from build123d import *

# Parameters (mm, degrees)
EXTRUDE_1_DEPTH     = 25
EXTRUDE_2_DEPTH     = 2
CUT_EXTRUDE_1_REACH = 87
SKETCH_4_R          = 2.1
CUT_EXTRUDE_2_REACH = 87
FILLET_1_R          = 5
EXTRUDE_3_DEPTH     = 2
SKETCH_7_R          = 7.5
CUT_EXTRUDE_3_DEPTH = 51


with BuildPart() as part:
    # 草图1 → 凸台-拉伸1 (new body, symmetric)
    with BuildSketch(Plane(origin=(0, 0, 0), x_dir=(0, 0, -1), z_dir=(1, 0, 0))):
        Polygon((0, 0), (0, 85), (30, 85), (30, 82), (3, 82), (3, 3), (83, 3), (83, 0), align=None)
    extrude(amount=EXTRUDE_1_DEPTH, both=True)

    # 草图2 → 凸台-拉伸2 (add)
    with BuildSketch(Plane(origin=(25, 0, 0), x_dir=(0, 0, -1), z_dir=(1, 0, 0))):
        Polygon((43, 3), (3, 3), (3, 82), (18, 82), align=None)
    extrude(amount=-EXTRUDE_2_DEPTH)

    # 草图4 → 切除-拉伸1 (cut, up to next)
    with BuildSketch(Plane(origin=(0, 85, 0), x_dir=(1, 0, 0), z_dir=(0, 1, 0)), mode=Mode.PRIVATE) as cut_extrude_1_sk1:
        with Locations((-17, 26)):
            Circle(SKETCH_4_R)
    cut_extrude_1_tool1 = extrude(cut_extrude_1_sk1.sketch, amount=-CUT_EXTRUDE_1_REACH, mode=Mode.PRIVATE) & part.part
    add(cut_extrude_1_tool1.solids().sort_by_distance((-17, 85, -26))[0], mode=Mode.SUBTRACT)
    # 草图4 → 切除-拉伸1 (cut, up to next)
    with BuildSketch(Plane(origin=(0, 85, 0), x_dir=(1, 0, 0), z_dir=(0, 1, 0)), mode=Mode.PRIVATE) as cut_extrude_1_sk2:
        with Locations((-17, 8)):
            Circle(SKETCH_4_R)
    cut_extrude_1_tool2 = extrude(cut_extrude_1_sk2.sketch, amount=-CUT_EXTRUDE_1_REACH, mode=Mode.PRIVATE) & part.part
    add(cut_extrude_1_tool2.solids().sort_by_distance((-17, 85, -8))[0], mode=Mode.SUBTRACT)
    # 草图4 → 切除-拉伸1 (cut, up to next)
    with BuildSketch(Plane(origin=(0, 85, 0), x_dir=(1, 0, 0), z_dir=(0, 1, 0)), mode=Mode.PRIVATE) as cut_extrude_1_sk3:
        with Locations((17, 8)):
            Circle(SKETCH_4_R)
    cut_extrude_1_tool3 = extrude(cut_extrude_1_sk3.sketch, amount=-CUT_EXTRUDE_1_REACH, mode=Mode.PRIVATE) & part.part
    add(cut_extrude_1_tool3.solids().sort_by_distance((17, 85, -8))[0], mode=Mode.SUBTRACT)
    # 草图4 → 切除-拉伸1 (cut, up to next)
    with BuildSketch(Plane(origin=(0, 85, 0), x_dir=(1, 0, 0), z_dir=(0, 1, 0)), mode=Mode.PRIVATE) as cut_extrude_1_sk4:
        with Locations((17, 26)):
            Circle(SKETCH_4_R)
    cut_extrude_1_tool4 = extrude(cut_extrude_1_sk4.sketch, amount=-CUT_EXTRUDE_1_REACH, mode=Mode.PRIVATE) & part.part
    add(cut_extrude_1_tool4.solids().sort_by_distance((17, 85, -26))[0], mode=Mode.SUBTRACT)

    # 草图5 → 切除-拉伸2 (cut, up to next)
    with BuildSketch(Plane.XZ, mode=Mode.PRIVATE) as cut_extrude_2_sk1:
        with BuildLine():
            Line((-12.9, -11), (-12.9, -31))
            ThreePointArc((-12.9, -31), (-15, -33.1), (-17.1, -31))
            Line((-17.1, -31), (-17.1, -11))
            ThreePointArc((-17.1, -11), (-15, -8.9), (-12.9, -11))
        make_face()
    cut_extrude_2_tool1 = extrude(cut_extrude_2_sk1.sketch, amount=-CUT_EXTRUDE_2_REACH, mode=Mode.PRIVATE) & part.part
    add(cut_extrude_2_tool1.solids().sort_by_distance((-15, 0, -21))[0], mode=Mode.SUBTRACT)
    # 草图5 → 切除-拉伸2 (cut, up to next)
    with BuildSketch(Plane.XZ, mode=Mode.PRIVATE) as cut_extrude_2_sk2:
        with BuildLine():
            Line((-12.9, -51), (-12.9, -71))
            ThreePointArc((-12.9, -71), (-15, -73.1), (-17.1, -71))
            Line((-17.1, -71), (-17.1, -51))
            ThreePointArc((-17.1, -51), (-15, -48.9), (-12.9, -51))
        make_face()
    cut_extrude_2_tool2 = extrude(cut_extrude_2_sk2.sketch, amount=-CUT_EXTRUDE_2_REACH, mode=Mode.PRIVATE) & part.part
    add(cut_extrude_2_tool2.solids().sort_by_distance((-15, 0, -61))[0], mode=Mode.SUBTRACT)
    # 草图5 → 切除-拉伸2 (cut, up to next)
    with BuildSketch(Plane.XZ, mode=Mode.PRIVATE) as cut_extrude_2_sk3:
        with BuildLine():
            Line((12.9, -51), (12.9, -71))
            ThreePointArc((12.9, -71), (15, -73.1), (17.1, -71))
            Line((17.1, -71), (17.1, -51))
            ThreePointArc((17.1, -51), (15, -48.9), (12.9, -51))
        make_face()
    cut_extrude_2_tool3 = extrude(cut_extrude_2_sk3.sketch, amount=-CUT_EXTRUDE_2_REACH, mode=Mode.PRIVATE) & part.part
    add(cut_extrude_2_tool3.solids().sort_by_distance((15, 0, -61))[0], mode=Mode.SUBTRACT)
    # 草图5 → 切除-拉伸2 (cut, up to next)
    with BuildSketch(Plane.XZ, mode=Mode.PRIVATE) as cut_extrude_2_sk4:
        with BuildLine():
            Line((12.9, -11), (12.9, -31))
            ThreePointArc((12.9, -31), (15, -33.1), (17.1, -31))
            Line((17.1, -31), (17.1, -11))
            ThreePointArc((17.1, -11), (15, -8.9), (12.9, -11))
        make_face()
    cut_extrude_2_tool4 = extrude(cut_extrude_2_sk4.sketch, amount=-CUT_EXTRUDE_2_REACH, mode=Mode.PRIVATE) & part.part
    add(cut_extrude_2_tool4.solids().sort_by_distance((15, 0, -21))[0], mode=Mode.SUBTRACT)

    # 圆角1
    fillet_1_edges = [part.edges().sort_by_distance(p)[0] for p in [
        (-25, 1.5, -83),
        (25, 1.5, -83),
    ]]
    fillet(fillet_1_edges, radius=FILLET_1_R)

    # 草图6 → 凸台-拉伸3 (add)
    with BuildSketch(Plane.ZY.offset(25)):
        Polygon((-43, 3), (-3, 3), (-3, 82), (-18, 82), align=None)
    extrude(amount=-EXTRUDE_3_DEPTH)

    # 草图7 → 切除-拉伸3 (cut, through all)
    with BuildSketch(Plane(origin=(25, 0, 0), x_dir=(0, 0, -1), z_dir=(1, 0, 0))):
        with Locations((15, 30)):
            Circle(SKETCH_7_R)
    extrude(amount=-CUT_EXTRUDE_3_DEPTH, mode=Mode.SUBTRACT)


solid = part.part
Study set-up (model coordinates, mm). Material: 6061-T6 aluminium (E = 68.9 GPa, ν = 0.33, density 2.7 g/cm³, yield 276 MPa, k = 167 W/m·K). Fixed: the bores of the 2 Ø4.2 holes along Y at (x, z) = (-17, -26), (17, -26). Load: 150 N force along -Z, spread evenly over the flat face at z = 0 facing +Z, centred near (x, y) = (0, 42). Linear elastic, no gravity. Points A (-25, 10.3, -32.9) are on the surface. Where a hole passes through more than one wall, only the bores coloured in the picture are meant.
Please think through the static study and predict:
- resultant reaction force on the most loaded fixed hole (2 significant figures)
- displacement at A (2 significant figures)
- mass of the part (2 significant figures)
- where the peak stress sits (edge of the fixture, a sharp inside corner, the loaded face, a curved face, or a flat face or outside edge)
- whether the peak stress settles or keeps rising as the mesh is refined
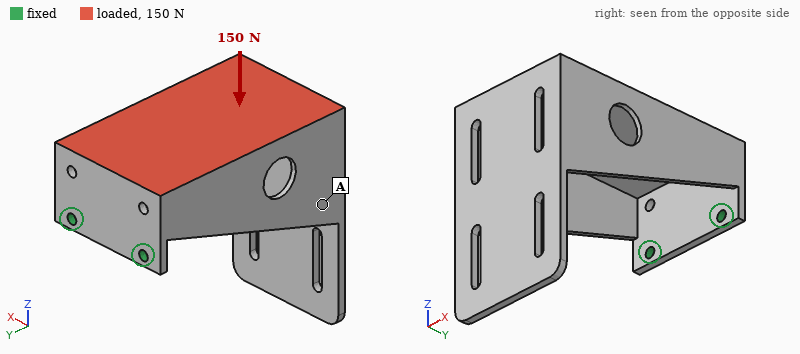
77 N
0.92 mm
96 g
edge of the fixture
keeps rising
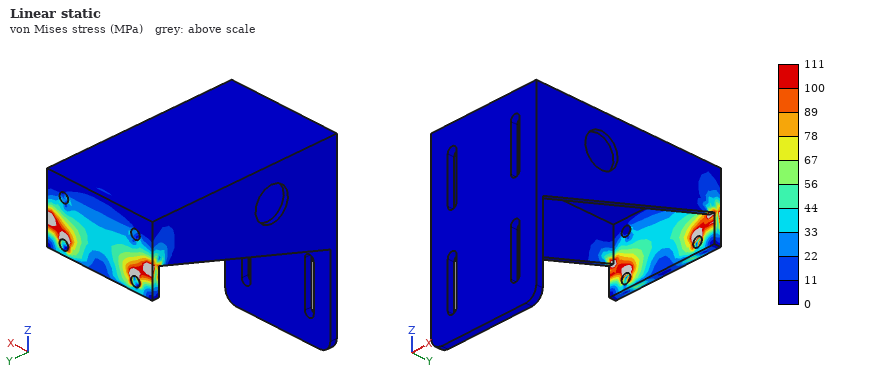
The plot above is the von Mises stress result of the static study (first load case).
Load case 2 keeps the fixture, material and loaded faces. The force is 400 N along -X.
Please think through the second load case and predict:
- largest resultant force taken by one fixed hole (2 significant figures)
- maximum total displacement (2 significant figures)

520 N
1.0 mm
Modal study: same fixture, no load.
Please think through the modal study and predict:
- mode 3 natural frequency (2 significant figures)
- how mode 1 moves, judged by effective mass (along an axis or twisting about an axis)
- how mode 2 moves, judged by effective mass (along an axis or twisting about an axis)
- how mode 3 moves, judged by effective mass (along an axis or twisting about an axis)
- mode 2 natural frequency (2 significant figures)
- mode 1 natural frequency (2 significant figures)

980 Hz
along Z
along X
along Y
250 Hz
180 Hz
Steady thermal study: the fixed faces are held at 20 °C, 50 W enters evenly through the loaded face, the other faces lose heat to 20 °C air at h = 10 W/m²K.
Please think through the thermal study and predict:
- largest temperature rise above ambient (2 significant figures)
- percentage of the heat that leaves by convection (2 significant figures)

69 K
26 %
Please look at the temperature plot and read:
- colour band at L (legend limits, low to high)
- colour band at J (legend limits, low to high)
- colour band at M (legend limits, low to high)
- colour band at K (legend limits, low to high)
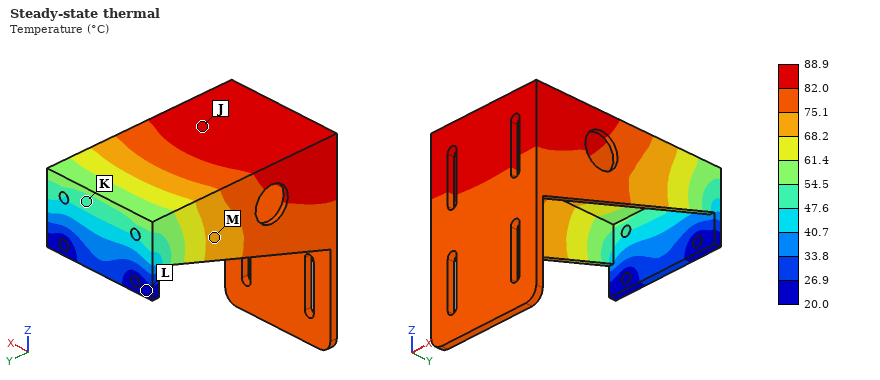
20.0 to 26.9 °C
82.0 to 88.9 °C
68.2 to 75.1 °C
47.6 to 54.5 °C
